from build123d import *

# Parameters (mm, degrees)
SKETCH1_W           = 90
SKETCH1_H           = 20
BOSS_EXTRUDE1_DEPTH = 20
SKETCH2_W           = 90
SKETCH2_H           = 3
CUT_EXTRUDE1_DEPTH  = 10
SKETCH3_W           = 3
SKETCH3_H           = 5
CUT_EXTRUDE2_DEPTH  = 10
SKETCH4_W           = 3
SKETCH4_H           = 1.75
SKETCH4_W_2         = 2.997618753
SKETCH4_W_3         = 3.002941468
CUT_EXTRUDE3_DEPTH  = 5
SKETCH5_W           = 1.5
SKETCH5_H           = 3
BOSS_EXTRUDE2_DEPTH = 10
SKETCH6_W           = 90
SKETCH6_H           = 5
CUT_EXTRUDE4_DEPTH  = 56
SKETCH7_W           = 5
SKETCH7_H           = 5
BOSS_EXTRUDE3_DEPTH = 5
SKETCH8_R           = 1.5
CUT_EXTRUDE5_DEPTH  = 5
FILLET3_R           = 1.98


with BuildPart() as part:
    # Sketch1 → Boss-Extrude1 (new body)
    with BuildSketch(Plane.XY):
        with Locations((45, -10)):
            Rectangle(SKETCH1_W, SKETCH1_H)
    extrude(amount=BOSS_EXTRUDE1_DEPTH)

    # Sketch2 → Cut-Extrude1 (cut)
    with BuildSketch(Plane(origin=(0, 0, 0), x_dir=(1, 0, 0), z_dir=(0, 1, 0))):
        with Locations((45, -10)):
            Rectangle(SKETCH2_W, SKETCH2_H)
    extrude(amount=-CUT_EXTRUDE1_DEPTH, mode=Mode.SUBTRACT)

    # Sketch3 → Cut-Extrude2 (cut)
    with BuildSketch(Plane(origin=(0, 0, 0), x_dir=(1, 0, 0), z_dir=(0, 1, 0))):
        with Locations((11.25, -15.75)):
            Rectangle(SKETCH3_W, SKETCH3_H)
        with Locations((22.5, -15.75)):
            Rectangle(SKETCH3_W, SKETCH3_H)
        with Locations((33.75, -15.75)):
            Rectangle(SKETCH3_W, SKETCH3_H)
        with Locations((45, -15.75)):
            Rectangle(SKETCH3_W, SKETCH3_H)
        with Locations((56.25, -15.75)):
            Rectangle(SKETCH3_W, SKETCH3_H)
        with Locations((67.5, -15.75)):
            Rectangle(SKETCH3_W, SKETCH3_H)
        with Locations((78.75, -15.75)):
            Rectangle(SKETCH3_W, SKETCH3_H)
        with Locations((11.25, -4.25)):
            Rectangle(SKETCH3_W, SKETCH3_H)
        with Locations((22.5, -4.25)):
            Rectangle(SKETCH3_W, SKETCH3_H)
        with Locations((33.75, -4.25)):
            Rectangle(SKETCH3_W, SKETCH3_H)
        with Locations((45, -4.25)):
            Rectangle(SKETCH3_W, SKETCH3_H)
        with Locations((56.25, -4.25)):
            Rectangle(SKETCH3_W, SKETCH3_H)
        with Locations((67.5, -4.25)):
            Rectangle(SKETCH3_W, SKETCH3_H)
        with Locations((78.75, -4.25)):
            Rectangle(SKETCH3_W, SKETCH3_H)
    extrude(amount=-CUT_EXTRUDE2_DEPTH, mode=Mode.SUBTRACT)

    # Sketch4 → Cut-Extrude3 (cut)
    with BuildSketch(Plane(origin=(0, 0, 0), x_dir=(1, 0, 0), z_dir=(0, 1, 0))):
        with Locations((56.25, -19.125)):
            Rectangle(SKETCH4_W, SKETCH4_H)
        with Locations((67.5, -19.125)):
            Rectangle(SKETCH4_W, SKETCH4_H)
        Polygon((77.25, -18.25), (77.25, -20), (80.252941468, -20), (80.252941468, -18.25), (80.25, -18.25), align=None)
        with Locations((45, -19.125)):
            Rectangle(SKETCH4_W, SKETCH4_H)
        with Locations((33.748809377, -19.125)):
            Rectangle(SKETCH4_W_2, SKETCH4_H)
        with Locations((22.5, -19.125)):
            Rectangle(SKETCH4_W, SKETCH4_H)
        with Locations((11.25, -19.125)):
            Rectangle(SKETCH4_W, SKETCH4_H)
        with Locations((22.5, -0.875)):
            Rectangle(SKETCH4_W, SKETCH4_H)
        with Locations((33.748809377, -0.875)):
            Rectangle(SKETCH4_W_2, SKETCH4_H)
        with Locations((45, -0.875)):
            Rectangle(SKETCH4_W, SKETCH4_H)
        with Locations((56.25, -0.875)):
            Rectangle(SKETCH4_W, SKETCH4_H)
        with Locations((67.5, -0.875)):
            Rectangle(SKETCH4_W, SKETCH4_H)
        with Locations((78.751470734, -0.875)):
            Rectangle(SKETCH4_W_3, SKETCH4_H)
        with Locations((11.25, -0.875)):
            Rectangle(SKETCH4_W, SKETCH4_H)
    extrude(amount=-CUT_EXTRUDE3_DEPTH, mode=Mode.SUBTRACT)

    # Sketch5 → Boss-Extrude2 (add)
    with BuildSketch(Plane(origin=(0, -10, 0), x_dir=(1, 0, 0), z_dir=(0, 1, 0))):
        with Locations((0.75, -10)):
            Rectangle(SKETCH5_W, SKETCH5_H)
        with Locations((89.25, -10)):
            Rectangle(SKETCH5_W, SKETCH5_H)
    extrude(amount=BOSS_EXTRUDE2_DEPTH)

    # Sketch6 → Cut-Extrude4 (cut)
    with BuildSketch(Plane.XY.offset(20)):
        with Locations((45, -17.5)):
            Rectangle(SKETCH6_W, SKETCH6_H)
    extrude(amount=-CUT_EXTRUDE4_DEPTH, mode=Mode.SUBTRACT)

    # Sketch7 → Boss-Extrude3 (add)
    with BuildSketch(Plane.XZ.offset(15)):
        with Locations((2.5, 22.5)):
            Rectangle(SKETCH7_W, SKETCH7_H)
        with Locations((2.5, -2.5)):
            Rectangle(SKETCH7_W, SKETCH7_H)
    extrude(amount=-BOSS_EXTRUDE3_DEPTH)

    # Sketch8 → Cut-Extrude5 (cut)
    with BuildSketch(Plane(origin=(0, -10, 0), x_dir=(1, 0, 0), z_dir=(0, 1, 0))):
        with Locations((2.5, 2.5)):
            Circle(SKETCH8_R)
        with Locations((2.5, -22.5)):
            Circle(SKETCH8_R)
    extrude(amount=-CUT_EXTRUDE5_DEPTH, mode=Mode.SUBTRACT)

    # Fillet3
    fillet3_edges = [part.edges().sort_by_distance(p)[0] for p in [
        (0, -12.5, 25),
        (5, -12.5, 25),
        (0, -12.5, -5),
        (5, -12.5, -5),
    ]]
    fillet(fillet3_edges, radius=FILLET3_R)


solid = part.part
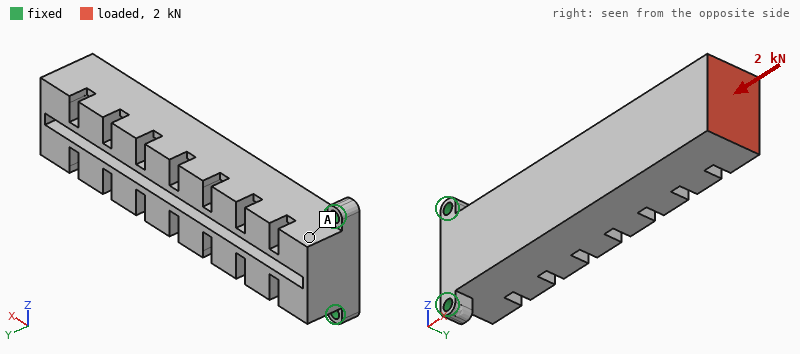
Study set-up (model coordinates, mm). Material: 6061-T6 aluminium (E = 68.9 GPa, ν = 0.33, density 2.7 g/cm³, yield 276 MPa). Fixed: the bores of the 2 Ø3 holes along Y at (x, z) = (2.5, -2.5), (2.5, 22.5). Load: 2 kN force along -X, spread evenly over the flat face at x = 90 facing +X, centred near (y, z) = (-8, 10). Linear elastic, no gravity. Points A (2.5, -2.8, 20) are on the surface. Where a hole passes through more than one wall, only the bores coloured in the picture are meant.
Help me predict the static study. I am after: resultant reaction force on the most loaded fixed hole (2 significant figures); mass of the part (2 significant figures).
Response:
1.1 kN
60 g
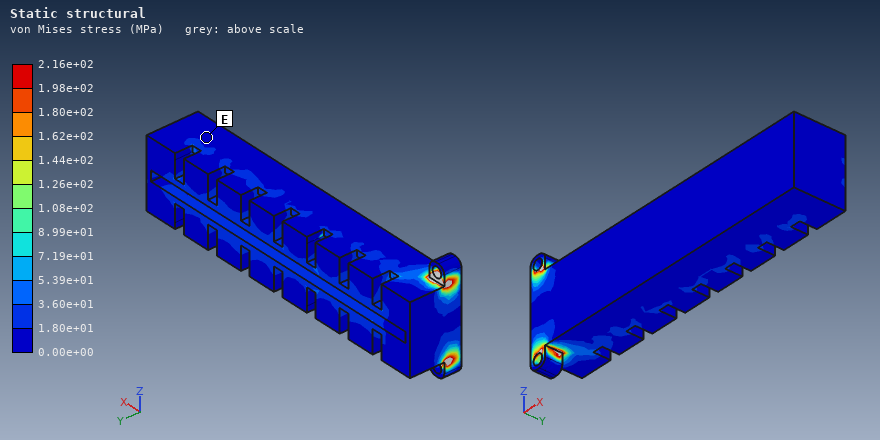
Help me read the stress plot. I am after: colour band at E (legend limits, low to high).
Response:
0.00e+00 to 1.80e+01 MPa
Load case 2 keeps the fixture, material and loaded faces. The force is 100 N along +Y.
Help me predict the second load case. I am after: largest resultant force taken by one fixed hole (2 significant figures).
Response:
58 N
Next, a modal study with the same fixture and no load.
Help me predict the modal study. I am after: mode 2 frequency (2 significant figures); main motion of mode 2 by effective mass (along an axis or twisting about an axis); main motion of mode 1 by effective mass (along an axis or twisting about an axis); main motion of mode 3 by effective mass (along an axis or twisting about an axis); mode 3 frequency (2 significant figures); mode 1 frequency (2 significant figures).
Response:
1400 Hz
along Z
along Y
twisting about X
4300 Hz
480 Hz
